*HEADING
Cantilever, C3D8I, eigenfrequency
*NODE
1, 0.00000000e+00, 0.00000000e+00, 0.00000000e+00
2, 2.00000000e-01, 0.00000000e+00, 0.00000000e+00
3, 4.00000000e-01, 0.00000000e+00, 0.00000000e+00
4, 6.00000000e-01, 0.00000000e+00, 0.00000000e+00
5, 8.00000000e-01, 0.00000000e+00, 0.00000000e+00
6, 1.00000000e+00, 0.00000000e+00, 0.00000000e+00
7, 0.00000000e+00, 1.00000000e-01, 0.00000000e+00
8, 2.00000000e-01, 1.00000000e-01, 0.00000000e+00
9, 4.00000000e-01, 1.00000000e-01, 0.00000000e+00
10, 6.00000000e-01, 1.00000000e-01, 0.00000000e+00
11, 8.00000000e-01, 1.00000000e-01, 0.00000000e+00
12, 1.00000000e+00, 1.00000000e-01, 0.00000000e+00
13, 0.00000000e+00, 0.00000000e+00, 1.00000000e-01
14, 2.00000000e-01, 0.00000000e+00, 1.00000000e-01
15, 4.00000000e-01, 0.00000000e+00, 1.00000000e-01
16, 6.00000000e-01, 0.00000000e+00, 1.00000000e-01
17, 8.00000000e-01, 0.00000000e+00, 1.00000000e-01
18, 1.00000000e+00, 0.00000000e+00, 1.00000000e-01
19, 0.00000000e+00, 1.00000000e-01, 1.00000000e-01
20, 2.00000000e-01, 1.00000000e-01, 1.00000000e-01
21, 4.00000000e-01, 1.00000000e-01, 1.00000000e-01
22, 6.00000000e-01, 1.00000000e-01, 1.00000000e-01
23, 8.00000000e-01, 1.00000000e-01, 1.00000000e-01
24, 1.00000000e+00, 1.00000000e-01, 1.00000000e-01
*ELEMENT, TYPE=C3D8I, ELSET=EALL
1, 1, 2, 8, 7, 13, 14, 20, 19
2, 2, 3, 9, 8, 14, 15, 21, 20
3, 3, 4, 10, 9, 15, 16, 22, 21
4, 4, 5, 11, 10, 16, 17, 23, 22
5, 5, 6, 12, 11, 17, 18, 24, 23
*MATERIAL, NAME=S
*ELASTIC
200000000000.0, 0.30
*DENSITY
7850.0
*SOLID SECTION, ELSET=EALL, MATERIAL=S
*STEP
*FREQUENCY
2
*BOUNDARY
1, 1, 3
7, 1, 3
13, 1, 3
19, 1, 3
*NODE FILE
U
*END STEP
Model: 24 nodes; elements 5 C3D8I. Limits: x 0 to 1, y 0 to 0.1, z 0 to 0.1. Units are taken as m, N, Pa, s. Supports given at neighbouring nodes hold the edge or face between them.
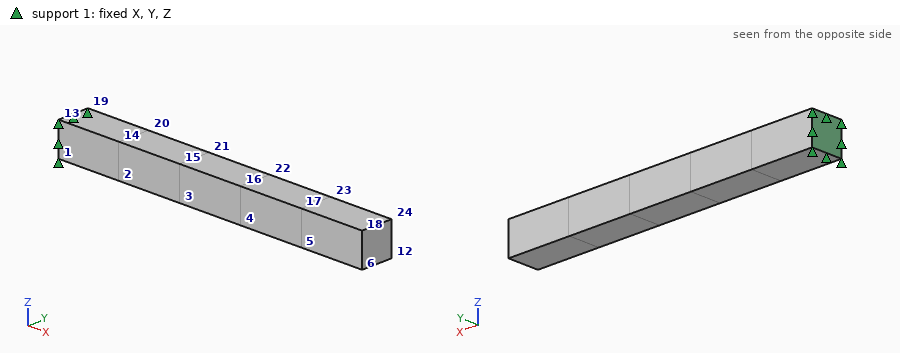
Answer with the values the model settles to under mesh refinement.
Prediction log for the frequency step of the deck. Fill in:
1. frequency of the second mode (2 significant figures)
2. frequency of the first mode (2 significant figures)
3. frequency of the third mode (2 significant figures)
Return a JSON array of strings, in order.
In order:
["83 Hz", "83 Hz", "500 Hz"]
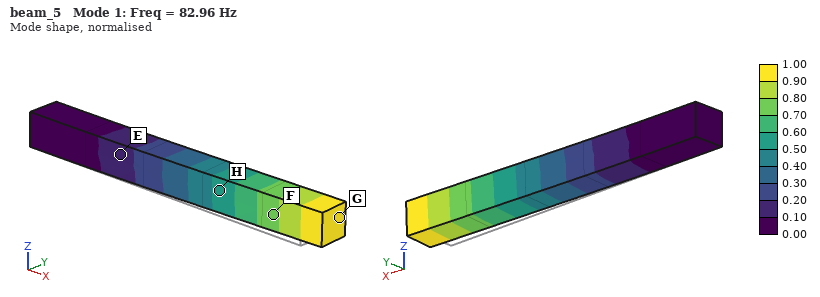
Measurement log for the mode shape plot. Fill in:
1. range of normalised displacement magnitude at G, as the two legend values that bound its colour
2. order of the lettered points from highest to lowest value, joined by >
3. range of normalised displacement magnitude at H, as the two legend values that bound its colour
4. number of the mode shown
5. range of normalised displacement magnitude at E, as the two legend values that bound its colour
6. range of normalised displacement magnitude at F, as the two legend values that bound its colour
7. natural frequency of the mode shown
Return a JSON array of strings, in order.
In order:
["0.90 to 1.00", "G > F > H > E", "0.50 to 0.60", "1", "0.10 to 0.20", "0.70 to 0.80", "82.96 Hz"]
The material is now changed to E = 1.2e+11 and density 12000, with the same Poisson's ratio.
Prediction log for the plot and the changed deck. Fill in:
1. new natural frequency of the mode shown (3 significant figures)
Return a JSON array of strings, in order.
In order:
["52.0 Hz"]
